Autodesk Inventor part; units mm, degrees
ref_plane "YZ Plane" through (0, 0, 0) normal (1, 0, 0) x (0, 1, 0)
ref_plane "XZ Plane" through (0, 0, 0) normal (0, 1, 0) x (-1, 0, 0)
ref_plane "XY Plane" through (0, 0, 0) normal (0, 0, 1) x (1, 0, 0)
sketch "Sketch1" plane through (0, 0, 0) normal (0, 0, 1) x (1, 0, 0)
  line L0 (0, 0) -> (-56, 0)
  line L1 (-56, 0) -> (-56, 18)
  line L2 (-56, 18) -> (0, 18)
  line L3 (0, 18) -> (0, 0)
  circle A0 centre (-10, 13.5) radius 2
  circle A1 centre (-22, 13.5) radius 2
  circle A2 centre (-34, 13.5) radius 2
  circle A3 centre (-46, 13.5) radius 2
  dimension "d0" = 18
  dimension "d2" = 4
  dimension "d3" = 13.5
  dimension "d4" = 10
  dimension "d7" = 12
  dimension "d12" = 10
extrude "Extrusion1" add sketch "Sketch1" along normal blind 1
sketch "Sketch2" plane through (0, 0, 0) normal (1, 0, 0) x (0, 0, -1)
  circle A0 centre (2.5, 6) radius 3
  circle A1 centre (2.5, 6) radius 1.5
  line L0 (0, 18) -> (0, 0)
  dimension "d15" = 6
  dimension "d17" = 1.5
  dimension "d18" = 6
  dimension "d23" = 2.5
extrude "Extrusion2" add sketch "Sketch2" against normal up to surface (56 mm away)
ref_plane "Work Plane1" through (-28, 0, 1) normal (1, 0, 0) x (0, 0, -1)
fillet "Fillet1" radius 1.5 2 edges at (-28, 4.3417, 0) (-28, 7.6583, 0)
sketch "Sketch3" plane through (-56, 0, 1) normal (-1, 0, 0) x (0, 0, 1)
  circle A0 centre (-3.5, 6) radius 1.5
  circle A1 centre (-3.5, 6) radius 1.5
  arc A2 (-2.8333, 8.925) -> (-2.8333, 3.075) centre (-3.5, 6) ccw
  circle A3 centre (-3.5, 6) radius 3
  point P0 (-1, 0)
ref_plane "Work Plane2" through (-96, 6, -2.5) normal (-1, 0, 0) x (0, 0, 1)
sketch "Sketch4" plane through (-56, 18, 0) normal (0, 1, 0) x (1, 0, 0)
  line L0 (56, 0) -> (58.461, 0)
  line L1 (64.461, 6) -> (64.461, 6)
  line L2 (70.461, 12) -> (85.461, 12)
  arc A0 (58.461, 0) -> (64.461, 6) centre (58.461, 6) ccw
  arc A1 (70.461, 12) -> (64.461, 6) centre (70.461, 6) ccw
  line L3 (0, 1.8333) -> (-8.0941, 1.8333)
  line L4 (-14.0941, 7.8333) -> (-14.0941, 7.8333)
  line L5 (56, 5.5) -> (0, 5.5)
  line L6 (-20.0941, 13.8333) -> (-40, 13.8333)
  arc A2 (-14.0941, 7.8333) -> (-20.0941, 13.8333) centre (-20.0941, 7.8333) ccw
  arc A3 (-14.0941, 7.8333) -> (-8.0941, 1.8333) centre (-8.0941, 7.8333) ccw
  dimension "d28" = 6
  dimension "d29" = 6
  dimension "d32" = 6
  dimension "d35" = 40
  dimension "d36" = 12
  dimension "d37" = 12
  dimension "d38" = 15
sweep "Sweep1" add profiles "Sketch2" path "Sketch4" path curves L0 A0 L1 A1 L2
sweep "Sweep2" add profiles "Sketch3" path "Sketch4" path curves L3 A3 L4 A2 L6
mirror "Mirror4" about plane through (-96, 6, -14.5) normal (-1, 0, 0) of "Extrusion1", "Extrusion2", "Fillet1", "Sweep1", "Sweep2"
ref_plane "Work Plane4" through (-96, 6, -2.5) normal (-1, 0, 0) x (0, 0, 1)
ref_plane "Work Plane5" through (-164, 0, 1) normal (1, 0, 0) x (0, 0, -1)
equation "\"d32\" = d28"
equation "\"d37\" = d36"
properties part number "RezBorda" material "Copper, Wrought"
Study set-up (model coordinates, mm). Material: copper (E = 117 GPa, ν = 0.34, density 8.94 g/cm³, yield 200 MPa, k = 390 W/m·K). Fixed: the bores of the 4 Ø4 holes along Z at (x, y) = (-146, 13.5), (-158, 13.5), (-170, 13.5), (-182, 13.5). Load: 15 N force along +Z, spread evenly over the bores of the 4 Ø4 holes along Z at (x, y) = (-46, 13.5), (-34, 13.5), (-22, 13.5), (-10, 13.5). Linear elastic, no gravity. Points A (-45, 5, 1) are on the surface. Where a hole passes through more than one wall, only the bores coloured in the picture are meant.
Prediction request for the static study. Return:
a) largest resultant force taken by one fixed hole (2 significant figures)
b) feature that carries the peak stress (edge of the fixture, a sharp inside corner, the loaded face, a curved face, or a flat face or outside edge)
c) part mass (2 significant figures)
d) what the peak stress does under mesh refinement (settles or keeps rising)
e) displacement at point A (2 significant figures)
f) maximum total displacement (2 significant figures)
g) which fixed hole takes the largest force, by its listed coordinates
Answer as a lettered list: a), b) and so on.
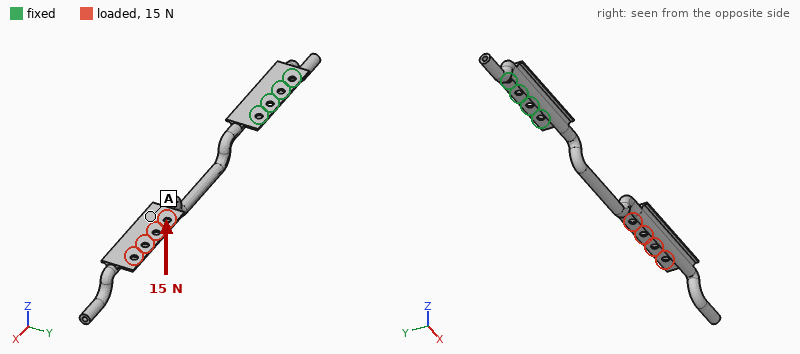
a) 130 N
b) edge of the fixture
c) 71 g
d) keeps rising
e) 1.1 mm
f) 2.4 mm
g) (-146, 13.5)
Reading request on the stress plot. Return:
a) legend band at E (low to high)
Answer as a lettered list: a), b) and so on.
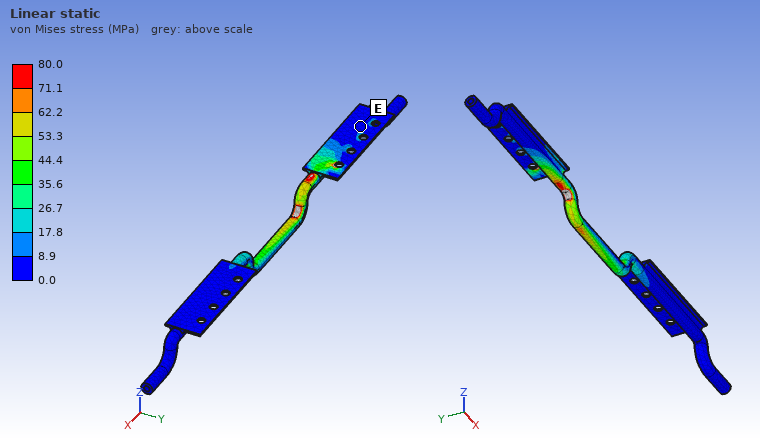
a) 0.0 to 8.9 MPa
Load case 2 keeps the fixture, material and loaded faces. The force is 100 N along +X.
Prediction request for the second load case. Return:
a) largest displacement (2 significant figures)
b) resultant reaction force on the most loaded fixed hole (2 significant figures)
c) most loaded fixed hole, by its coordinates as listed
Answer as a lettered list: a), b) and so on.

a) 2.4 mm
b) 85 N
c) (-146, 13.5)
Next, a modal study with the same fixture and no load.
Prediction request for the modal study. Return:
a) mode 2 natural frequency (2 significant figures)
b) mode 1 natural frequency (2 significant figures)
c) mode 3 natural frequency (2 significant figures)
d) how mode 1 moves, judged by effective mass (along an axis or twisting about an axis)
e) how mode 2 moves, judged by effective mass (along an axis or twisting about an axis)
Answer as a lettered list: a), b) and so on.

a) 87 Hz
b) 83 Hz
c) 570 Hz
d) along Z
e) along Y
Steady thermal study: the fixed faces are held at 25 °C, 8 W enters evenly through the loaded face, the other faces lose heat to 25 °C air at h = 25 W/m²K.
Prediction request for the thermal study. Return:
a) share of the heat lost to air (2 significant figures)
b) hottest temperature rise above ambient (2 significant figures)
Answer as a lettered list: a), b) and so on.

a) 68 %
b) 45 K
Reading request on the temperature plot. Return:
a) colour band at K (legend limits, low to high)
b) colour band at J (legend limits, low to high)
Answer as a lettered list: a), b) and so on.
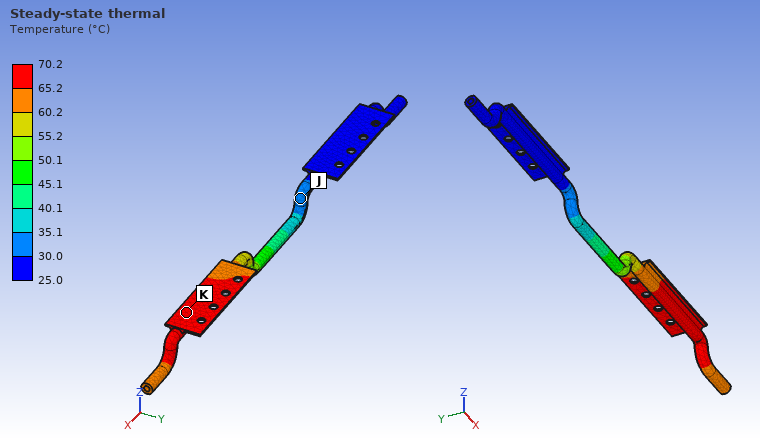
a) 65.2 to 70.2 °C
b) 30.0 to 35.1 °C
